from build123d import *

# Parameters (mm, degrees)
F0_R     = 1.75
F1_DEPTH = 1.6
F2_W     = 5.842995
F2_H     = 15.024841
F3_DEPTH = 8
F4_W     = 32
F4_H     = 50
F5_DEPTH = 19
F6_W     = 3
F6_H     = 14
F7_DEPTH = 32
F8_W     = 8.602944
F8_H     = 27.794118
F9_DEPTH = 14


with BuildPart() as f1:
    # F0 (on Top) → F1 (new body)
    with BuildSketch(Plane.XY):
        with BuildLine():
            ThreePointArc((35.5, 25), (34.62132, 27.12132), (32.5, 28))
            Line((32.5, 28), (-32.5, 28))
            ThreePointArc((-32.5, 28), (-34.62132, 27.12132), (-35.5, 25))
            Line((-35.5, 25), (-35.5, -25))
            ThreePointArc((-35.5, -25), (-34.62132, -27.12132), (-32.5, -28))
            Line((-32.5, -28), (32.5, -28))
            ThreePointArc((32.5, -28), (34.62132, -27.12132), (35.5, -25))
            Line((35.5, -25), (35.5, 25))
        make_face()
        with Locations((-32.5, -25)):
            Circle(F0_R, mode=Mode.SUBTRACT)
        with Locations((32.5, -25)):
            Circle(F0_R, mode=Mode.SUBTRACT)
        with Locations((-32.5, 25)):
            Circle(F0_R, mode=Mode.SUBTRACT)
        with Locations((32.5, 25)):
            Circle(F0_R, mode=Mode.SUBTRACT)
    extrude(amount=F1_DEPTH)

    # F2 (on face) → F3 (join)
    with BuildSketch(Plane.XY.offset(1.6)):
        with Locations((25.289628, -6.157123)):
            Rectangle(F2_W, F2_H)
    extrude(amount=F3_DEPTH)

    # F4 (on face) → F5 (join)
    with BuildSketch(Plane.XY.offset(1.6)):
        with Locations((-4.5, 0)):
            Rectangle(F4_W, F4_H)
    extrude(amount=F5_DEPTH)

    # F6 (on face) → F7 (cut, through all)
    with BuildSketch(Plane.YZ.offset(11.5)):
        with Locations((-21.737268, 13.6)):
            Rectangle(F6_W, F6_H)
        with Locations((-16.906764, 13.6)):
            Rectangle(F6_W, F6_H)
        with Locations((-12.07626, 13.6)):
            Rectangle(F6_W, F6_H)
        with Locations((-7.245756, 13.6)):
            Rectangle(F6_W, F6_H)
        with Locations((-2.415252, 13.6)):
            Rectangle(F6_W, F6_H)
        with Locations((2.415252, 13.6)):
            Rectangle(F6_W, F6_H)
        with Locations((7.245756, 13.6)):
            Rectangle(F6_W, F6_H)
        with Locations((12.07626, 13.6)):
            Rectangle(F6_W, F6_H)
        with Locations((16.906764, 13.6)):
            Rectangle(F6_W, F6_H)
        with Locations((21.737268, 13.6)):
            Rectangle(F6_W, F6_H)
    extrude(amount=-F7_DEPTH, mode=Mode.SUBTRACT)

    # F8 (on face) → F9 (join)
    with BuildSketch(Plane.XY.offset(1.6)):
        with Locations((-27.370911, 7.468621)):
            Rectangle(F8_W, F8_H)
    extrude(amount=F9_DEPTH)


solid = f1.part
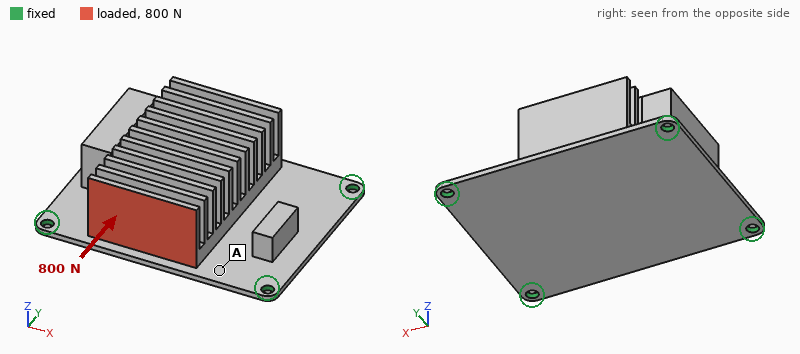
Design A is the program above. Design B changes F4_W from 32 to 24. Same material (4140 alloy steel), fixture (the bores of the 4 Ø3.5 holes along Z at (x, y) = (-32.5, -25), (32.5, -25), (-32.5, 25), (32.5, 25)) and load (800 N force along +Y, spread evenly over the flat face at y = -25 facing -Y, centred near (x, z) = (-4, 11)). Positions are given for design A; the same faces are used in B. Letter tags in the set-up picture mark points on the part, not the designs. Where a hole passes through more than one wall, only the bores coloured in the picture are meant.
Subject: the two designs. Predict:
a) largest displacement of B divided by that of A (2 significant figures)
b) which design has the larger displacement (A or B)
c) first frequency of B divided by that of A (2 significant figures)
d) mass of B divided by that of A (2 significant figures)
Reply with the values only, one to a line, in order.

1.5
B
0.89
0.84
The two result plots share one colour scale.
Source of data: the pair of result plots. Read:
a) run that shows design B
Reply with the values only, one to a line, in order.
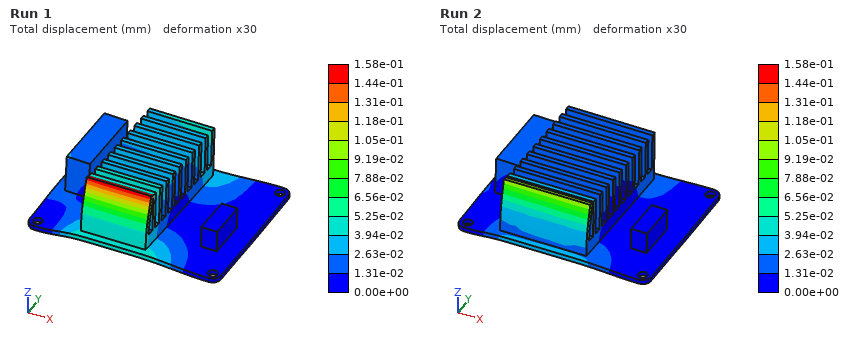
Run 1
